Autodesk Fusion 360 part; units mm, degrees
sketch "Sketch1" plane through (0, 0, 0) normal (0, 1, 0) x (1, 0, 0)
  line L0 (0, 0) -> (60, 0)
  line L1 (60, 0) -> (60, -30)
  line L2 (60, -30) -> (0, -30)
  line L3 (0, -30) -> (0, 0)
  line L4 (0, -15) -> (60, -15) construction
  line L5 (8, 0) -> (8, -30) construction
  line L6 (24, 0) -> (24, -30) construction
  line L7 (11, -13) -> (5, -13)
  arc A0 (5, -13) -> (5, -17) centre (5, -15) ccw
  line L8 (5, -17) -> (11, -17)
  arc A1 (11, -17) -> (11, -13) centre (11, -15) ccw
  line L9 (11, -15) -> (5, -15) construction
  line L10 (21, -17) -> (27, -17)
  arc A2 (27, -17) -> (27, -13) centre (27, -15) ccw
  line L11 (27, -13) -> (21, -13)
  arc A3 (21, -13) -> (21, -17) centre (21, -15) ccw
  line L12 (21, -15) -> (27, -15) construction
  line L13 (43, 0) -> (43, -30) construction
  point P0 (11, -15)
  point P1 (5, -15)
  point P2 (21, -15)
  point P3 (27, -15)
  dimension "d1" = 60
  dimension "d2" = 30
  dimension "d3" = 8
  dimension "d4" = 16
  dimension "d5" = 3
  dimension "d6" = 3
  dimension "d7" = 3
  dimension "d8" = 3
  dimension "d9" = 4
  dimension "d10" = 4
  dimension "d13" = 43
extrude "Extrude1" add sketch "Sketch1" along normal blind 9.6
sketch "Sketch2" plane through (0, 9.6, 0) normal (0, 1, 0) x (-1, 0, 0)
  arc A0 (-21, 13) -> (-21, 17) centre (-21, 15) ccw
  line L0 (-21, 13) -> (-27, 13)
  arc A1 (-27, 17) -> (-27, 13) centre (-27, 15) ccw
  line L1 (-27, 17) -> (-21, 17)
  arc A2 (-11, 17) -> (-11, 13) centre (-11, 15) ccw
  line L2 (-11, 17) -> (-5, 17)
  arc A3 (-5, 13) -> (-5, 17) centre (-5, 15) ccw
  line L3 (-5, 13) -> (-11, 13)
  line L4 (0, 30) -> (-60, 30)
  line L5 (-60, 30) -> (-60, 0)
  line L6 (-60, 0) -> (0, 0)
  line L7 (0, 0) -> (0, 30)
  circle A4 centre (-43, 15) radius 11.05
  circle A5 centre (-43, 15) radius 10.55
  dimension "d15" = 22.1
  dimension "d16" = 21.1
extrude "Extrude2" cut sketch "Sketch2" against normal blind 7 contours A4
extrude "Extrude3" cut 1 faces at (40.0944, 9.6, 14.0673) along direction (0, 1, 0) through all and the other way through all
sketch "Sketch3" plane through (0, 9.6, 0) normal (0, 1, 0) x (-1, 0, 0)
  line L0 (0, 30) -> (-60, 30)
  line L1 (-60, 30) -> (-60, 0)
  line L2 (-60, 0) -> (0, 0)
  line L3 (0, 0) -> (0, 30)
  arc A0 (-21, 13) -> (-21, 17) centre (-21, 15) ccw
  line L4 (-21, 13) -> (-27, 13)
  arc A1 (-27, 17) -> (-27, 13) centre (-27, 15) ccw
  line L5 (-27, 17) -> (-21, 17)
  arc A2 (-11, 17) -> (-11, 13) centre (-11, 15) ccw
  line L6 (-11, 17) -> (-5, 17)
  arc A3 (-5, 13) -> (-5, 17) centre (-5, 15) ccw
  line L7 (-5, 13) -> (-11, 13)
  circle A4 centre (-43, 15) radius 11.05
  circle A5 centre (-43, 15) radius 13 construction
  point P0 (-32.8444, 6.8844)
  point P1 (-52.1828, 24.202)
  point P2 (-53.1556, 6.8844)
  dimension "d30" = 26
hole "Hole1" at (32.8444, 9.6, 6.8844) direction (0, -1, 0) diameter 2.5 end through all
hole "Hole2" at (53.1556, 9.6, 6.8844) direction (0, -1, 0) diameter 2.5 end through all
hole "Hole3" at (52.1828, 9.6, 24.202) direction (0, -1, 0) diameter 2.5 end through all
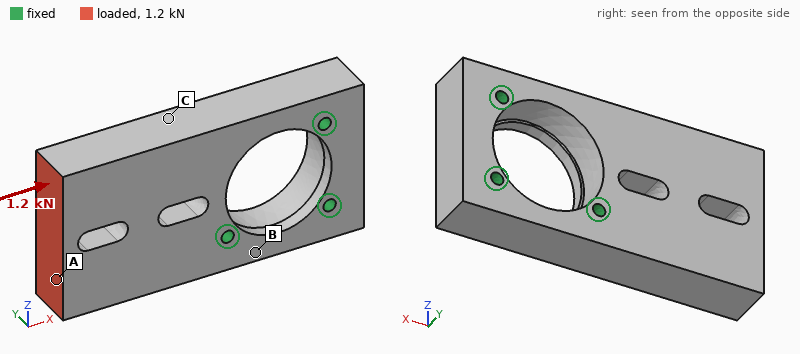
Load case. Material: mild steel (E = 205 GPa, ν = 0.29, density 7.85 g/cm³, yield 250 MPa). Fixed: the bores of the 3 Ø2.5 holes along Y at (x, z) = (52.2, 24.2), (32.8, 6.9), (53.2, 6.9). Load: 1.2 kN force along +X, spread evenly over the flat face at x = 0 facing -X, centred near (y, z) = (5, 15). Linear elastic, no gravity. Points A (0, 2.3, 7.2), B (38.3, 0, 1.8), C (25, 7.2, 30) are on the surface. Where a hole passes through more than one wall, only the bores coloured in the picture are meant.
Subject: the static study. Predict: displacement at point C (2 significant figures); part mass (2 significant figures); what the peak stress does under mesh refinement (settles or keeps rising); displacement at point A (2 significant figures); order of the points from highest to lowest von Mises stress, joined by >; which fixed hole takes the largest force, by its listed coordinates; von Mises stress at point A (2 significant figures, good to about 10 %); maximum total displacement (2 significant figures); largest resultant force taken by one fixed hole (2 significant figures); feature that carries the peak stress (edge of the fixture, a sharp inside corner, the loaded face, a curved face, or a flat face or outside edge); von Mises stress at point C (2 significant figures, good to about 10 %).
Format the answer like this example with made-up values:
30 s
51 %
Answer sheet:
1.6 µm
100 g
keeps rising
1.9 µm
C > A > B
(32.8, 6.9)
4.7 MPa
2.8 µm
730 N
edge of the fixture
8.4 MPa
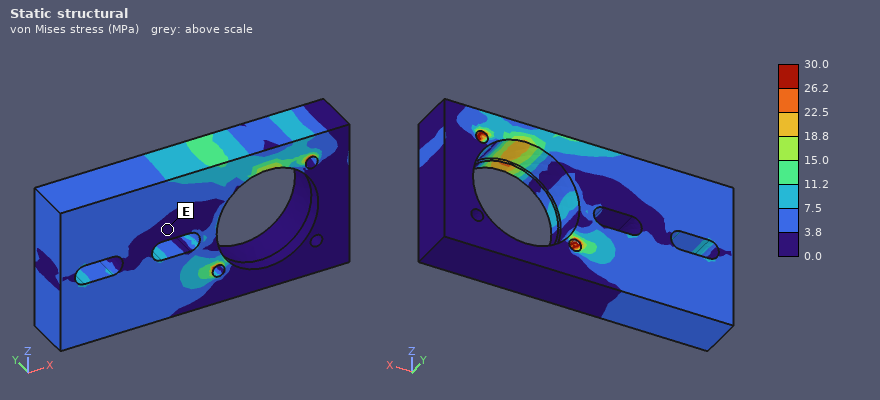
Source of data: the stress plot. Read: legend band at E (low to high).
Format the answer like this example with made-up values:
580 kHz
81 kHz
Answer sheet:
0.0 to 3.8 MPa
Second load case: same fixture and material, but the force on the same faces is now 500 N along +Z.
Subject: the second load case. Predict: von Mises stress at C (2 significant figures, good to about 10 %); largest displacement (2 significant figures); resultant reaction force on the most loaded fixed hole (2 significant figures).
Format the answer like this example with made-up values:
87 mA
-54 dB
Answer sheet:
13 MPa
6.9 µm
740 N
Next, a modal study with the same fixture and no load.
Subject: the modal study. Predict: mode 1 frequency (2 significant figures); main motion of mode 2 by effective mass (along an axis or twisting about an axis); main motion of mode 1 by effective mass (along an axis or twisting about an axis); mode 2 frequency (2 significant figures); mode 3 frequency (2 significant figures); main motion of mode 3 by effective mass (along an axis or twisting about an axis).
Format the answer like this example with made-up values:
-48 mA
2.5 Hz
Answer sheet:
4300 Hz
along Z
along Y
8800 Hz
9800 Hz
twisting about X
